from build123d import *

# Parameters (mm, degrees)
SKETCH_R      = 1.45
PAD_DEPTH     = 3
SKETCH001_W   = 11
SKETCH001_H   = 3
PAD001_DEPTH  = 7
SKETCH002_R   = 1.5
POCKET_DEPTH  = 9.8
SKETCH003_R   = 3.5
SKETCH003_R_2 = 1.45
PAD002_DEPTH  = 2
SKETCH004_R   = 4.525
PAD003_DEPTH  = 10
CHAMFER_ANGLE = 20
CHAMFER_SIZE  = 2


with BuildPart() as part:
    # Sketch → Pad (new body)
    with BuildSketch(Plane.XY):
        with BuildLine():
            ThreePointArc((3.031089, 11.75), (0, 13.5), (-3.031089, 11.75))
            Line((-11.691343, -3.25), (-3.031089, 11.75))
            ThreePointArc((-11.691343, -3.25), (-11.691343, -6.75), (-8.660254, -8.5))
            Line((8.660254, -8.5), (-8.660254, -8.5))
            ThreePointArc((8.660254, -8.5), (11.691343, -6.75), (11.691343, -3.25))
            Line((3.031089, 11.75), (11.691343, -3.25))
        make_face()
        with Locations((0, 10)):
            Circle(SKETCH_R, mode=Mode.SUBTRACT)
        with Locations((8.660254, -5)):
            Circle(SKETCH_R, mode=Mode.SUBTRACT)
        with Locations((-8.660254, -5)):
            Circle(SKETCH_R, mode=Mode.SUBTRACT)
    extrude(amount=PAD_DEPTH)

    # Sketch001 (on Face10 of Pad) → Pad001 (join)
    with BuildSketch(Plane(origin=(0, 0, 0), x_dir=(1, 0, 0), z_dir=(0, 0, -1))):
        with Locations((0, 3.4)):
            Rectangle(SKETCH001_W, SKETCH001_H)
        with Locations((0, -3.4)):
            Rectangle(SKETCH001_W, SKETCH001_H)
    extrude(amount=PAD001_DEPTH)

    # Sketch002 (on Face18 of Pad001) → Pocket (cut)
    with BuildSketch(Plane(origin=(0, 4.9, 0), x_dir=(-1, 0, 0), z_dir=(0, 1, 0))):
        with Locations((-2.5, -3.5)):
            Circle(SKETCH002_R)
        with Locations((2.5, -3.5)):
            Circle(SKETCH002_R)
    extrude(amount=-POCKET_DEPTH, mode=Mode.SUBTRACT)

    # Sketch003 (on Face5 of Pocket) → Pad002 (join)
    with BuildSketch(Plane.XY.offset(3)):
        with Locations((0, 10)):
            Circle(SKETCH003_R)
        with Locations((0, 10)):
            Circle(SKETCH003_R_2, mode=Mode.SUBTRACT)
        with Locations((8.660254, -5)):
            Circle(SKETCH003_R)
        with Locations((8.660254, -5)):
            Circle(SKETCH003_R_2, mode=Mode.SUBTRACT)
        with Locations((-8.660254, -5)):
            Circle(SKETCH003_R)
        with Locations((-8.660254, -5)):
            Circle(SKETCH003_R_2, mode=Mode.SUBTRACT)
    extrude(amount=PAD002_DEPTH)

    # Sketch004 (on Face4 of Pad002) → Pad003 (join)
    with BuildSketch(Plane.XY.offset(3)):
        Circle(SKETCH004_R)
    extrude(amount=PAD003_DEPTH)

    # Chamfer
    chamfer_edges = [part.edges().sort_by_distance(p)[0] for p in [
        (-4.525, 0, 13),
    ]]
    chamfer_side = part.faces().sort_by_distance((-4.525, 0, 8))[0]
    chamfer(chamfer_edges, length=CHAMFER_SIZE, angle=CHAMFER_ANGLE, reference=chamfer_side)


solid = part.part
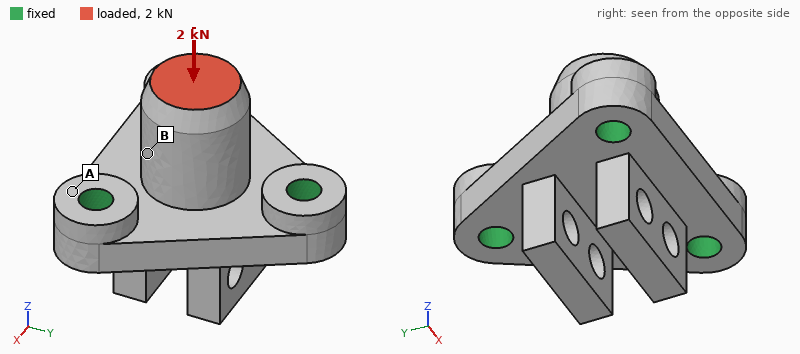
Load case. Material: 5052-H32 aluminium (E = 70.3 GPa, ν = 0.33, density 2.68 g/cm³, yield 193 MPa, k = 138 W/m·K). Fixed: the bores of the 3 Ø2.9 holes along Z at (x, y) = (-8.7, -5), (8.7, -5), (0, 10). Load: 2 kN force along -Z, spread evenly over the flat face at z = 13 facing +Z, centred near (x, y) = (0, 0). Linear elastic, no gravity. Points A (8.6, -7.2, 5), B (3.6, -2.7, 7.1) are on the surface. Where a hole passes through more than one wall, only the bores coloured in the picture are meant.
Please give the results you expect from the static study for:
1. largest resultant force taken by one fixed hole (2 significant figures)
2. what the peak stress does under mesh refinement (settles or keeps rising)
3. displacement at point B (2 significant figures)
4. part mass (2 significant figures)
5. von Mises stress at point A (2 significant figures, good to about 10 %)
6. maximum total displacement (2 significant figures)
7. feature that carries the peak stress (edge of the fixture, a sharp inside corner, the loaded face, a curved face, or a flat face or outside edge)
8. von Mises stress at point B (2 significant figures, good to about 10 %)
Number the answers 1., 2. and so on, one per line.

1. 690 N
2. keeps rising
3. 11 µm
4. 5.9 g
5. 14 MPa
6. 15 µm
7. edge of the fixture
8. 31 MPa
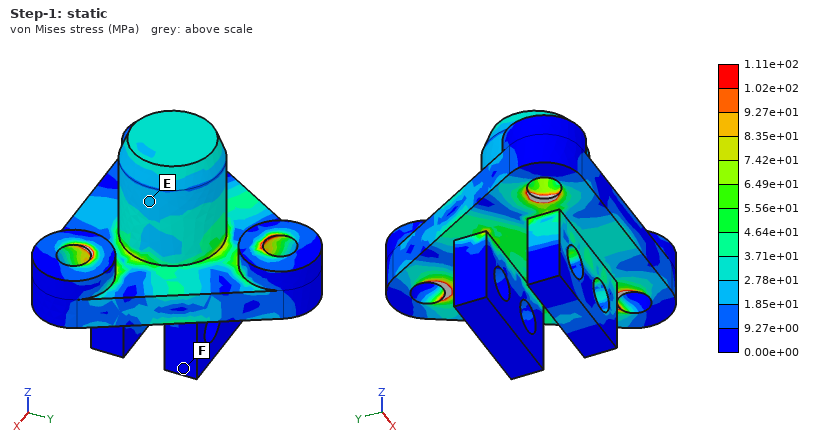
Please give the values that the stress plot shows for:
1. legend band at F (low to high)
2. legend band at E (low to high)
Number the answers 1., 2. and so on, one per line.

1. 0.00e+00 to 9.27e+00 MPa
2. 1.85e+01 to 2.78e+01 MPa
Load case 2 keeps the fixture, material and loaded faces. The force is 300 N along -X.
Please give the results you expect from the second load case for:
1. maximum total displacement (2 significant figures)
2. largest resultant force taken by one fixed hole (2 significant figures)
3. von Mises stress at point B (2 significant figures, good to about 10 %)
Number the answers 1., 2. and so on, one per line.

1. 16 µm
2. 250 N
3. 21 MPa
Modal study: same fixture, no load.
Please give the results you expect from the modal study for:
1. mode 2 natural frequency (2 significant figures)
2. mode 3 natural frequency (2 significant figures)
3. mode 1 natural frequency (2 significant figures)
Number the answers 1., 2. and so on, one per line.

1. 27 kHz
2. 31 kHz
3. 27 kHz
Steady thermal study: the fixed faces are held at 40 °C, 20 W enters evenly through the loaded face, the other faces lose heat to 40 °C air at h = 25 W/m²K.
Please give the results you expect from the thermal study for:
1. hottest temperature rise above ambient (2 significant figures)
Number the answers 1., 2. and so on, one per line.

1. 35 K
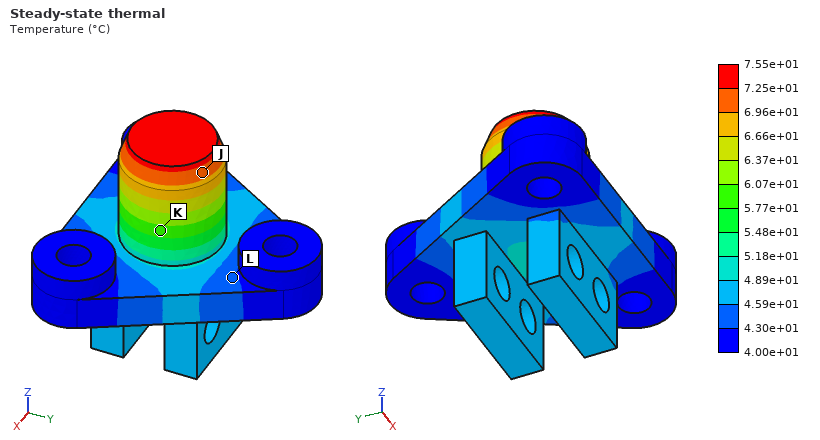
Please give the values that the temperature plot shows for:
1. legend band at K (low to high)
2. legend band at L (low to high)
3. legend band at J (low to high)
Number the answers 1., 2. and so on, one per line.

1. 5.77e+01 to 6.07e+01 °C
2. 4.30e+01 to 4.59e+01 °C
3. 6.96e+01 to 7.25e+01 °C
